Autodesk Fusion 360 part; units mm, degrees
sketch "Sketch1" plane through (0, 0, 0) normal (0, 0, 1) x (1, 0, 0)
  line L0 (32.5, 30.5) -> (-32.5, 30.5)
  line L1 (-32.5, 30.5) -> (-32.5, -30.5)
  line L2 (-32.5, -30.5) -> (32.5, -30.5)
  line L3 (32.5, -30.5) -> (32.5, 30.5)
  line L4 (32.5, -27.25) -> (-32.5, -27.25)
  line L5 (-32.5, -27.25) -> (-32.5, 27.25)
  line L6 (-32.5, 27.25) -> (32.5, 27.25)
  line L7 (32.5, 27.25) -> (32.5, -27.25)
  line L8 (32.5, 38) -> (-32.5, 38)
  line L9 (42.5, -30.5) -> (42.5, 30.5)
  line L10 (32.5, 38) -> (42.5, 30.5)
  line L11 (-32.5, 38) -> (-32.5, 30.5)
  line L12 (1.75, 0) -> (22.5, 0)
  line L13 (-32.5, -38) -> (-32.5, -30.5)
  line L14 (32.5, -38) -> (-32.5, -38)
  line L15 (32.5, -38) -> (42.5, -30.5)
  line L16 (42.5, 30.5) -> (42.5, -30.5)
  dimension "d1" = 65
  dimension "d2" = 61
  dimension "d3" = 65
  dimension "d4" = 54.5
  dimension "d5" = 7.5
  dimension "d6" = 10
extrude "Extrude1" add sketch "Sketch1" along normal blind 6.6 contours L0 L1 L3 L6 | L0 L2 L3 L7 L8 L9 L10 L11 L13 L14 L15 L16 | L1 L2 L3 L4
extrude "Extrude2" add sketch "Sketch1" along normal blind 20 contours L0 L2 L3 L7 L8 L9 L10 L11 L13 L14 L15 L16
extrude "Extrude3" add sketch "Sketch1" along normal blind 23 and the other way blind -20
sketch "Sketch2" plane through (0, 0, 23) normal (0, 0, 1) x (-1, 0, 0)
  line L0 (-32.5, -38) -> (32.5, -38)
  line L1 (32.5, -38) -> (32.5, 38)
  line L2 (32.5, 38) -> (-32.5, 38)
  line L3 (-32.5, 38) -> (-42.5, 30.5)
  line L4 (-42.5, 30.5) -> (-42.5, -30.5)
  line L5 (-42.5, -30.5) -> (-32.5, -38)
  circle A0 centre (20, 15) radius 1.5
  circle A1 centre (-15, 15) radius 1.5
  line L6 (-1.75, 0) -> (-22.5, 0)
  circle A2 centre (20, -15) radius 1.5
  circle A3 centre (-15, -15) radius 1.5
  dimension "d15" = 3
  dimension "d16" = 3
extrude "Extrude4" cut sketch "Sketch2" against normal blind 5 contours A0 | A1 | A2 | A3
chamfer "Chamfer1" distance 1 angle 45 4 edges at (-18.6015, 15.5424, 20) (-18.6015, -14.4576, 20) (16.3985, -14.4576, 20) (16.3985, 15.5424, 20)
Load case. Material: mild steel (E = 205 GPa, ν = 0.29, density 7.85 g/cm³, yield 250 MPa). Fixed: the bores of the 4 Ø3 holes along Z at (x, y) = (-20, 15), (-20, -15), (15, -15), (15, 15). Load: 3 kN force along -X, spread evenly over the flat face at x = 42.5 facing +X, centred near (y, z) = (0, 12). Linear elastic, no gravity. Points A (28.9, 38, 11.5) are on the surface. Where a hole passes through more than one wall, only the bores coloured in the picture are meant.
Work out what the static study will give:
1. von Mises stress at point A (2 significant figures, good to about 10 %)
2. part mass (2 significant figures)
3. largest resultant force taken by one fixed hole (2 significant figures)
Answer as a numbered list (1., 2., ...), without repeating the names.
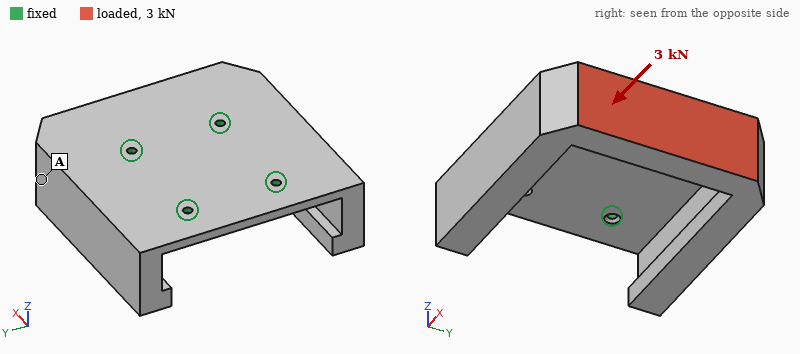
1. 14 MPa
2. 410 g
3. 1.1 kN
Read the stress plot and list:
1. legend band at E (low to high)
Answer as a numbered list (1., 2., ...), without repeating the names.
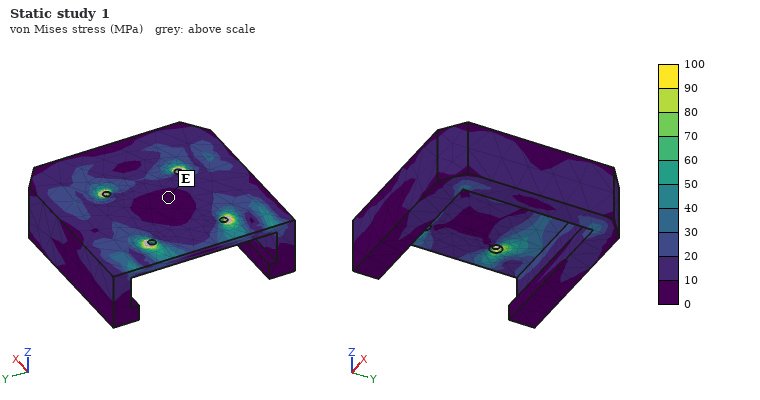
1. 0 to 10 MPa
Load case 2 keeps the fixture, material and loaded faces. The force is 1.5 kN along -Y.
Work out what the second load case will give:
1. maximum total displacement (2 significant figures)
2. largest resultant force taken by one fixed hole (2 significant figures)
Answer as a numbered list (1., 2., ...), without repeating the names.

1. 35 µm
2. 1.2 kN
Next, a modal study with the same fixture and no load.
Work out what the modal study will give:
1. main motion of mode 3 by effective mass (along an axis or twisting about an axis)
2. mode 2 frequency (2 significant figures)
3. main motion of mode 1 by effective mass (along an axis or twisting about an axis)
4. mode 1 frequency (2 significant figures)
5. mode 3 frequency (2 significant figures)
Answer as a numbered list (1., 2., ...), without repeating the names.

1. along Z
2. 1800 Hz
3. along Y
4. 1500 Hz
5. 2500 Hz
